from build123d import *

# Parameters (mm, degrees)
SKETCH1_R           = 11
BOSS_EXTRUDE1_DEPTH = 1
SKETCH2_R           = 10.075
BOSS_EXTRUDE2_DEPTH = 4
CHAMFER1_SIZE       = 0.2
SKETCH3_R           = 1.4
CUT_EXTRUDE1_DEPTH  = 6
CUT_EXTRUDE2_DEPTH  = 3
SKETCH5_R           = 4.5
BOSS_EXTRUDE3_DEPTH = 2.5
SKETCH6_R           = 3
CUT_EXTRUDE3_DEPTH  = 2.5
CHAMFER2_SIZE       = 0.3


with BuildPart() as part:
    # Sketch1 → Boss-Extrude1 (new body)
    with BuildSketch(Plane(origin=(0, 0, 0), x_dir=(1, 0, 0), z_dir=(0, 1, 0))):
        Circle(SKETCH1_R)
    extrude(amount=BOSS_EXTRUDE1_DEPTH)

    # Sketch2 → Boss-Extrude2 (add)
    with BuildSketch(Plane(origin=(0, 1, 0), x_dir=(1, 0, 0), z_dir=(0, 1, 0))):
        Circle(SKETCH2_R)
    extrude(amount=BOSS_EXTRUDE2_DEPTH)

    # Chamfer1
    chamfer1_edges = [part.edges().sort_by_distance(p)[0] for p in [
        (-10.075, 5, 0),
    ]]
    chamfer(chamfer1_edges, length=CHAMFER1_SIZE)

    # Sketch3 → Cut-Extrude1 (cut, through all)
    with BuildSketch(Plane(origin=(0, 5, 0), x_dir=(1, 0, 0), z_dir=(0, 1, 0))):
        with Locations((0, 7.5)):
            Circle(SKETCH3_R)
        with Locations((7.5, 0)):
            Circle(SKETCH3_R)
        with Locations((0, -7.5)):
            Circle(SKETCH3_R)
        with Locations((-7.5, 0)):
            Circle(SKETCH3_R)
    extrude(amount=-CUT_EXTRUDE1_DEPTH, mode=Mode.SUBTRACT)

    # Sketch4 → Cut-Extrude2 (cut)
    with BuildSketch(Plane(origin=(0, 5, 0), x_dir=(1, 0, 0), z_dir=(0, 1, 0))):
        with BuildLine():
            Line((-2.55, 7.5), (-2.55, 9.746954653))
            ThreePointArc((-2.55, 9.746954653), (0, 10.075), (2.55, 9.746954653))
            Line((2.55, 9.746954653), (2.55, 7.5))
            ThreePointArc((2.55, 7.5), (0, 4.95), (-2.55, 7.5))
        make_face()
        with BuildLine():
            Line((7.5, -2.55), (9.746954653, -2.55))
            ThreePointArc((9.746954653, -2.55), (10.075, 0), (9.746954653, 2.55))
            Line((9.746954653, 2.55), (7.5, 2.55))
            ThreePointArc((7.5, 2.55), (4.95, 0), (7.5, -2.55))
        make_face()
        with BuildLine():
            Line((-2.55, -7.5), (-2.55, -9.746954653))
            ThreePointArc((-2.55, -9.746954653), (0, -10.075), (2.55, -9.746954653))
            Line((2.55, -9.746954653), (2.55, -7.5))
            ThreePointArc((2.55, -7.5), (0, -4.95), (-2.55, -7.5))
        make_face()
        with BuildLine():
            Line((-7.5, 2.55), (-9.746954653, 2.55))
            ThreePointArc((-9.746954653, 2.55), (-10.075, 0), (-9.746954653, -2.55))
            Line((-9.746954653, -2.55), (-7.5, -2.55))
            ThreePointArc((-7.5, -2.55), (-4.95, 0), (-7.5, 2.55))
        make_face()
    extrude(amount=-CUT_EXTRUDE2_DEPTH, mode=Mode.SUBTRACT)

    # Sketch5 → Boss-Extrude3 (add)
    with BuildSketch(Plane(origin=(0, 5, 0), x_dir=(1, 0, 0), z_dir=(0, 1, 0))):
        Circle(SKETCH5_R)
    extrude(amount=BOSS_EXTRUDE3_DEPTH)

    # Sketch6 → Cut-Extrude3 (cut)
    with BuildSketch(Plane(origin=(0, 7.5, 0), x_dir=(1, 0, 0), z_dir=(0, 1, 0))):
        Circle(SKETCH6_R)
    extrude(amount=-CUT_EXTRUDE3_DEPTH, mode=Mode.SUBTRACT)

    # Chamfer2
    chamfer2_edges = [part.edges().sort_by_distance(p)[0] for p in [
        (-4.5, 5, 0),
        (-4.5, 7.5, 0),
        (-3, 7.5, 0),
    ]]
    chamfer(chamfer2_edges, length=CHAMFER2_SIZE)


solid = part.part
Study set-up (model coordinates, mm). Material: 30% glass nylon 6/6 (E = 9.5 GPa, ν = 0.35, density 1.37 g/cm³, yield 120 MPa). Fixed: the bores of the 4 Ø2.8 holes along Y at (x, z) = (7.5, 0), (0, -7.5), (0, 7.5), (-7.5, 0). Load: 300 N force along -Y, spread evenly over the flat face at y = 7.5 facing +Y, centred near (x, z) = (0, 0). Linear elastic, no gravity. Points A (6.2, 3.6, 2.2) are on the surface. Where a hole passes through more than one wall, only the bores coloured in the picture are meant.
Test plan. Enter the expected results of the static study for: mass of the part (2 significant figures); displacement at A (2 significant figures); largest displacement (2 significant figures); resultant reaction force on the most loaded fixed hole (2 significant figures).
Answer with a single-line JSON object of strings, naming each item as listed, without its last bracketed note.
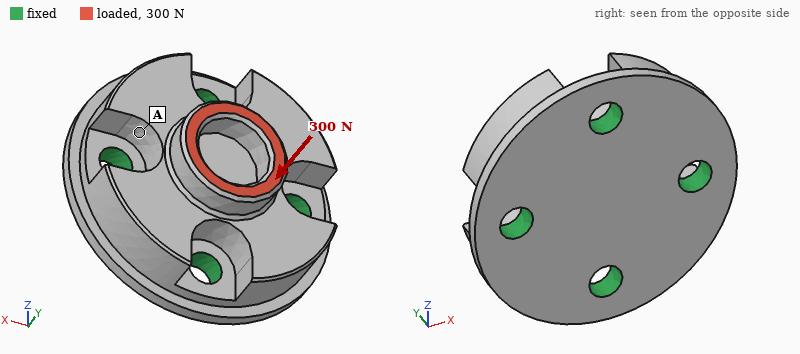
{"mass of the part": "1.9 g", "displacement at A": "3.0 µm", "largest displacement": "7.7 µm", "resultant reaction force on the most loaded fixed hole": "81 N"}
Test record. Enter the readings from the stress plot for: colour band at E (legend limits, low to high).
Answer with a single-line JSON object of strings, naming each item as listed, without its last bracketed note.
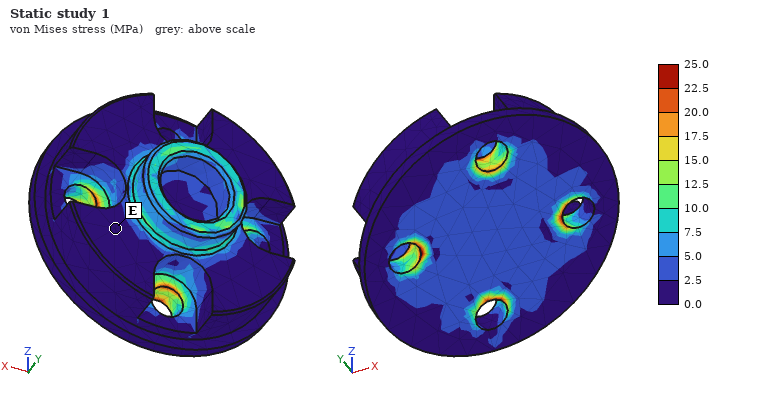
{"colour band at E": "0.0 to 2.5 MPa"}
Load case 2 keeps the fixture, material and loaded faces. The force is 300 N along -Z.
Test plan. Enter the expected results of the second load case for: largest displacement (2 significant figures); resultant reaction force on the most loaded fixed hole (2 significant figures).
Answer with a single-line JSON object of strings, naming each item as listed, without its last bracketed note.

{"largest displacement": "32 µm", "resultant reaction force on the most loaded fixed hole": "160 N"}
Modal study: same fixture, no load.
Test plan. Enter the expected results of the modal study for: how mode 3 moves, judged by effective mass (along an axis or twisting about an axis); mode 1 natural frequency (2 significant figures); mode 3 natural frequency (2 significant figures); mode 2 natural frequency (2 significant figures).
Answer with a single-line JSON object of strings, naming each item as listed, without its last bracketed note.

{"how mode 3 moves, judged by effective mass": "along Y", "mode 1 natural frequency": "32 kHz", "mode 3 natural frequency": "36 kHz", "mode 2 natural frequency": "32 kHz"}
